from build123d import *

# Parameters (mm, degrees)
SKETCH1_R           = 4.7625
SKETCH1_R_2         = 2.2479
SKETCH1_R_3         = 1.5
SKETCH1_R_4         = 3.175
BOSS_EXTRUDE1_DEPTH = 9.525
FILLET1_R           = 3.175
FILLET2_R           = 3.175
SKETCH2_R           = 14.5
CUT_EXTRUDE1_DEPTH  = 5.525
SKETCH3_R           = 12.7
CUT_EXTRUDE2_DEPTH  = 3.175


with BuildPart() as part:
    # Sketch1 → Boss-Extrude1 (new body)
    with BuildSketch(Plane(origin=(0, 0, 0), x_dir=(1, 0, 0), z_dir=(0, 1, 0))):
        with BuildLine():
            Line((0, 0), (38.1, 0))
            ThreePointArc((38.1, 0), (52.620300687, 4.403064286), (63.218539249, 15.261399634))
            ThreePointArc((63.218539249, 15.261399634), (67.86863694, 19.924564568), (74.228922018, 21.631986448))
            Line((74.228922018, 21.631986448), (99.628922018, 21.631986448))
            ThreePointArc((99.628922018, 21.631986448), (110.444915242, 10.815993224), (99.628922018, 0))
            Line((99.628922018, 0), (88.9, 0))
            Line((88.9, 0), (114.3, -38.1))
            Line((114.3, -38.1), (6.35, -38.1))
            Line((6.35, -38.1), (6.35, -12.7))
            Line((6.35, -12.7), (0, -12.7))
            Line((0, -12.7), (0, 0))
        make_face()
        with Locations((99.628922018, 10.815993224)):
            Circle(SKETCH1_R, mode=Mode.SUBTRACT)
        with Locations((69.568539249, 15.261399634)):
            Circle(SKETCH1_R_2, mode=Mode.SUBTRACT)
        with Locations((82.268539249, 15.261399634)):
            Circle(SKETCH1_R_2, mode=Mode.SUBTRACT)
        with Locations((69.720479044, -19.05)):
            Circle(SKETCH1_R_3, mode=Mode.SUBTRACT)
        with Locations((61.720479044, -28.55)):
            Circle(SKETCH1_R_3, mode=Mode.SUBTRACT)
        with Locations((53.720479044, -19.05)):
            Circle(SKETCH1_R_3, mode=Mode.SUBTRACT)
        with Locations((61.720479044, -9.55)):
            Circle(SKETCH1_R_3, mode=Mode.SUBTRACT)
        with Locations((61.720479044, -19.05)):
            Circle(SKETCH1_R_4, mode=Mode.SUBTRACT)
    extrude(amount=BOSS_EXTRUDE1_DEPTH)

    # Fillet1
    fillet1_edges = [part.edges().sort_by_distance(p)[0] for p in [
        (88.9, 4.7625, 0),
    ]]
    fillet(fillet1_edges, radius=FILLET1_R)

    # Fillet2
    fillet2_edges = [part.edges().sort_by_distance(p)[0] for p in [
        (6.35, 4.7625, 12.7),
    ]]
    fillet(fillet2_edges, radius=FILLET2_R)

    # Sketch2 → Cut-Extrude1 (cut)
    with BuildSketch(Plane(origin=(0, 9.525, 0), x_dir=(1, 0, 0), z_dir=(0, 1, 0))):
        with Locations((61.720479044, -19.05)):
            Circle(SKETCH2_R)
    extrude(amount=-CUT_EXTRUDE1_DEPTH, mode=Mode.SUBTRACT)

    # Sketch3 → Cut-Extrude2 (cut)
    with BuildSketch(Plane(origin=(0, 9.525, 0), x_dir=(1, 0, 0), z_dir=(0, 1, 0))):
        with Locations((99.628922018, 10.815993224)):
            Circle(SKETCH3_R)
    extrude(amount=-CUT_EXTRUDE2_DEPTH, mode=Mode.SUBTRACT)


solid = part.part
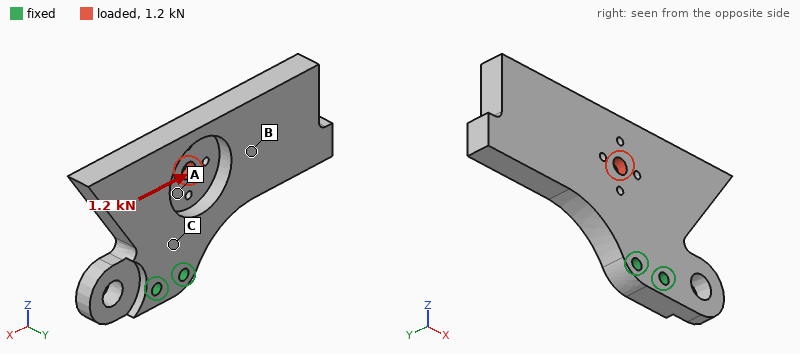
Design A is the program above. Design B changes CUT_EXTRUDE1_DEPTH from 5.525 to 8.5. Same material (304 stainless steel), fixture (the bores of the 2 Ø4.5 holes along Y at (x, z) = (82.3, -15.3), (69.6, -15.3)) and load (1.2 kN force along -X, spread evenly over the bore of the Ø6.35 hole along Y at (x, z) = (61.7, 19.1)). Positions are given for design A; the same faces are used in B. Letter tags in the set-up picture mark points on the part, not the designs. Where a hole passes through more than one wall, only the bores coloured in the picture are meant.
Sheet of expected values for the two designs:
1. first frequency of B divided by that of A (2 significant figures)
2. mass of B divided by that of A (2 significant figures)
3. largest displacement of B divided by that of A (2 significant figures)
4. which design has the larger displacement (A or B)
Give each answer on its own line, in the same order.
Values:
0.99
0.95
1.3
B
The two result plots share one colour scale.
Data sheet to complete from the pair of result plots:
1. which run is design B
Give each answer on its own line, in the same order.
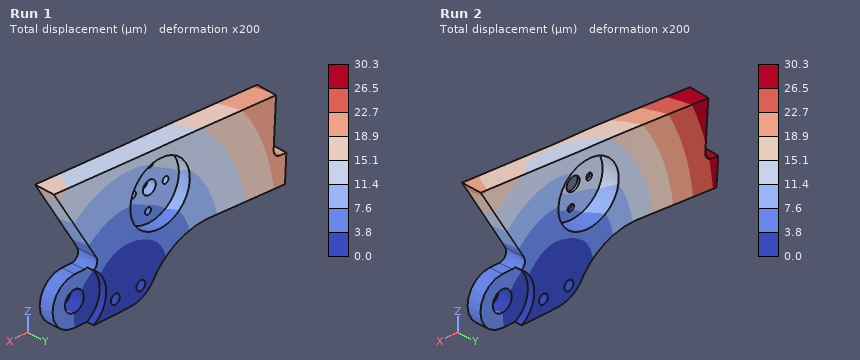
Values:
Run 2
